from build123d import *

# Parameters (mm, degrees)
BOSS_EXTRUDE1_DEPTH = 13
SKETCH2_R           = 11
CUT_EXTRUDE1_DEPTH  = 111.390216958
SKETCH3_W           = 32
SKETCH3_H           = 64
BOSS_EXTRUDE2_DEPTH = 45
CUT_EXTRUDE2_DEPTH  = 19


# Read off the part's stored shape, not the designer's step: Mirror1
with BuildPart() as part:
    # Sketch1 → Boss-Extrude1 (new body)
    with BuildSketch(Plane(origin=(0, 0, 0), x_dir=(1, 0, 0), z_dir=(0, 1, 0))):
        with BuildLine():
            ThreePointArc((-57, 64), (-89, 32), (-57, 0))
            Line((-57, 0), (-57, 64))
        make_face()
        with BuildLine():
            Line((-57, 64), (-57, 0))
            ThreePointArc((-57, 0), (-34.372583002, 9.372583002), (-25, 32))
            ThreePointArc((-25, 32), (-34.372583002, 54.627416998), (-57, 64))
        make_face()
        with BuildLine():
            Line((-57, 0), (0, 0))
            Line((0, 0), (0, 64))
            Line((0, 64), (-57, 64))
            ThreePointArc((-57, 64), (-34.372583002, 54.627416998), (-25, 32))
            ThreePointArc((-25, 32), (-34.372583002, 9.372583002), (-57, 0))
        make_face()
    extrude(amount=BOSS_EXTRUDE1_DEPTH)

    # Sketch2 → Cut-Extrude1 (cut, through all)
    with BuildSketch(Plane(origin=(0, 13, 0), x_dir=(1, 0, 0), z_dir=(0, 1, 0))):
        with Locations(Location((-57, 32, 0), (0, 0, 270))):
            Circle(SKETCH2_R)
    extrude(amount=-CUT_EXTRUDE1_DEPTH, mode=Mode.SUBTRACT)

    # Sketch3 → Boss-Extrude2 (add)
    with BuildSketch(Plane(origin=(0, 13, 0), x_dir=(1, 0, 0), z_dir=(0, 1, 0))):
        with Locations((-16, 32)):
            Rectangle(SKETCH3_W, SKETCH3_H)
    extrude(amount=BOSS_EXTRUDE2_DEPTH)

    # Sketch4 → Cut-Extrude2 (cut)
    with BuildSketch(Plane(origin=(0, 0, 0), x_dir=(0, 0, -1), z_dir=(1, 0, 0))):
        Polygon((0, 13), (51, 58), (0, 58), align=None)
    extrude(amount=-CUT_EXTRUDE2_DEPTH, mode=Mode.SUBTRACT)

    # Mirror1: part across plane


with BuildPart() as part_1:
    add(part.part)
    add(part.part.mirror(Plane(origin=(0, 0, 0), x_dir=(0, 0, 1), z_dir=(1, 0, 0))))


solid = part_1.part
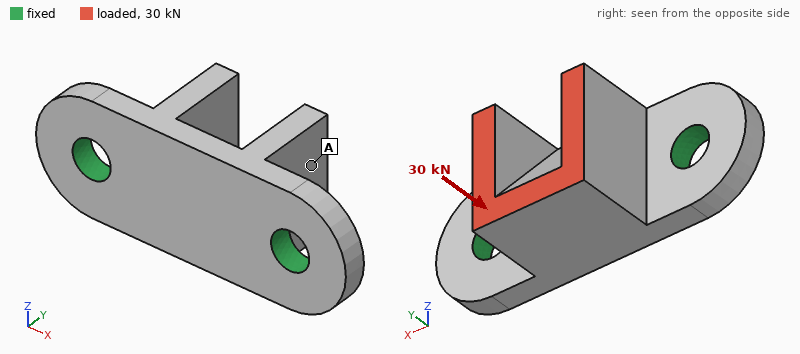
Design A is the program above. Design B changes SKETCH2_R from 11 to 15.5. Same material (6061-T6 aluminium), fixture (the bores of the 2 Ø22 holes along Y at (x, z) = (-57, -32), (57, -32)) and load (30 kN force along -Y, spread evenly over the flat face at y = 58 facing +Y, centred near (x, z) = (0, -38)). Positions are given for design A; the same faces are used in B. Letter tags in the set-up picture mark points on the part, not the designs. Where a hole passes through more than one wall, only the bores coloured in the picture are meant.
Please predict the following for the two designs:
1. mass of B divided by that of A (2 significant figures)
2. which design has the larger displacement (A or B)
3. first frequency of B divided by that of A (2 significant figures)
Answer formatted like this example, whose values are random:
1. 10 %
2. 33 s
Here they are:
1. 0.96
2. A
3. 1.2
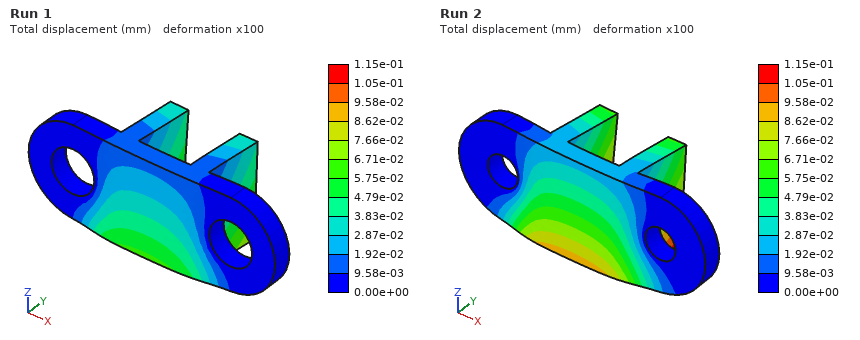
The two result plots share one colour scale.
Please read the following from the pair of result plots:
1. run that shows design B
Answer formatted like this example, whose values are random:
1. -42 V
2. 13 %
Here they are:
1. Run 1
